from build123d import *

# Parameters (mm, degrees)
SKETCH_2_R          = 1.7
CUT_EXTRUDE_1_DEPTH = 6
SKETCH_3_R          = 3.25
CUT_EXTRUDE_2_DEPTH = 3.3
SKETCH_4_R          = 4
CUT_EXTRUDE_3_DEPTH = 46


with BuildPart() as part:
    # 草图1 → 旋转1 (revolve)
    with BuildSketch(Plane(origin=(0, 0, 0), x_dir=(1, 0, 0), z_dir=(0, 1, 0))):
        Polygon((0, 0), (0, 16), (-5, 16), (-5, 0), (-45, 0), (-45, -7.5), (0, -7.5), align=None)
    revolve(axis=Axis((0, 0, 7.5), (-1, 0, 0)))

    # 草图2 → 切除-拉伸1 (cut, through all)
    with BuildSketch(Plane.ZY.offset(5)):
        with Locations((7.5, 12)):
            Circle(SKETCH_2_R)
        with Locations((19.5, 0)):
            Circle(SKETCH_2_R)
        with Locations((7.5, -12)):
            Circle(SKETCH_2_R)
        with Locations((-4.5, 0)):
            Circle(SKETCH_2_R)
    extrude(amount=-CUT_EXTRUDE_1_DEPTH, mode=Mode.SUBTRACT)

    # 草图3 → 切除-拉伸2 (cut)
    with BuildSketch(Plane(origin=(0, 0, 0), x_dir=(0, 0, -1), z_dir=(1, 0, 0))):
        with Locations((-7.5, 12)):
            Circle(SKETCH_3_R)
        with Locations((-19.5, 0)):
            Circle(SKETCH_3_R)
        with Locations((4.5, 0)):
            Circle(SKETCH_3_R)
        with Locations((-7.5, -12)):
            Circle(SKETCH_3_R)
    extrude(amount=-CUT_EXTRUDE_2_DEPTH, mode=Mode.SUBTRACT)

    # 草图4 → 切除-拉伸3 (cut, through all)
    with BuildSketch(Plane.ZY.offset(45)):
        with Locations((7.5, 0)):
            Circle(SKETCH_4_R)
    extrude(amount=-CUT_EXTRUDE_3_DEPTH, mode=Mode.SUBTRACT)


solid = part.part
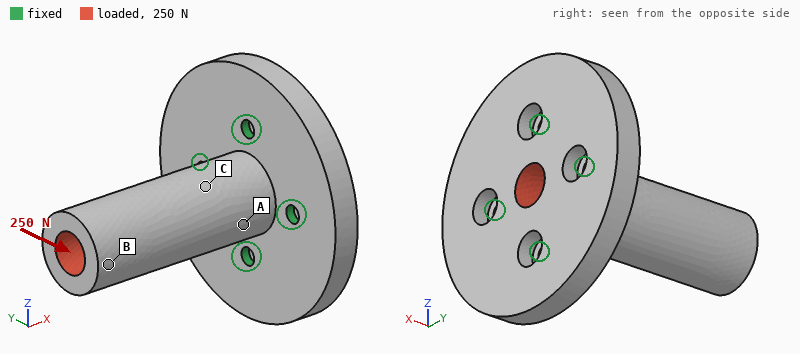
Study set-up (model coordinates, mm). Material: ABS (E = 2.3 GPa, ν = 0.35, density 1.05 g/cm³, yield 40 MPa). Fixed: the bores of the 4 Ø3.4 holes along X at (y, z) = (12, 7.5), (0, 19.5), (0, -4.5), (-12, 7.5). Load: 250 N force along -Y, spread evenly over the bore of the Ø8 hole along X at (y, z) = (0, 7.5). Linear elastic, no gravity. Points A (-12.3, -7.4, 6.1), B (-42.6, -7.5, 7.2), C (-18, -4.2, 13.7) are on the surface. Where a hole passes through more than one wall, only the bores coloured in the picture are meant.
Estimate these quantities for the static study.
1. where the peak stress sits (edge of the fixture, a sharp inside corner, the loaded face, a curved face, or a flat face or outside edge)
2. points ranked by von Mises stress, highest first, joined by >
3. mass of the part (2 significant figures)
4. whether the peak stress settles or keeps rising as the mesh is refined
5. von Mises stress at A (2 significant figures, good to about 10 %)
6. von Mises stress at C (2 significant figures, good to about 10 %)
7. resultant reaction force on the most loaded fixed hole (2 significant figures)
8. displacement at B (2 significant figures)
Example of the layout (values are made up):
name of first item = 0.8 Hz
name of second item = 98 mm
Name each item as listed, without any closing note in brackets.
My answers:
where the peak stress sits = edge of the fixture
points ranked by von Mises stress, highest first, joined by > = A > C > B
mass of the part = 14 g
whether the peak stress settles or keeps rising as the mesh is refined = keeps rising
von Mises stress at A = 9.1 MPa
von Mises stress at C = 4.6 MPa
resultant reaction force on the most loaded fixed hole = 200 N
displacement at B = 0.76 mm
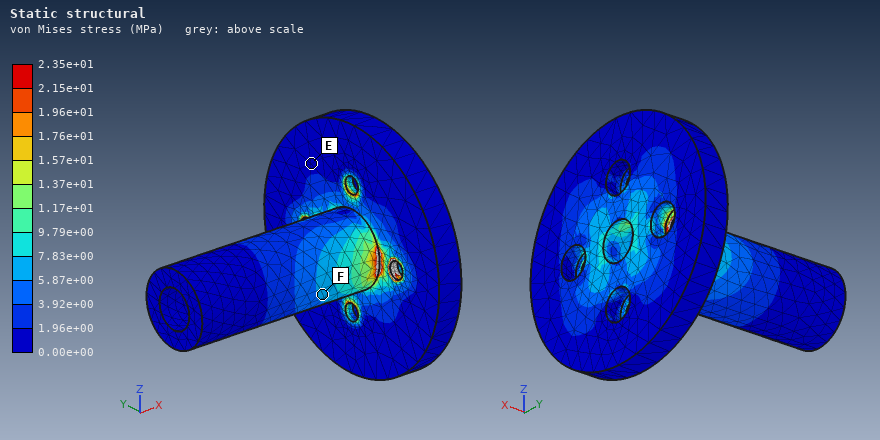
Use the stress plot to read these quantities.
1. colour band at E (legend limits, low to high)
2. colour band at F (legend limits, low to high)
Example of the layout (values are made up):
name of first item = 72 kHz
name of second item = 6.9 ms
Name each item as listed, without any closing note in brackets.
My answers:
colour band at E = 0.00e+00 to 1.96e+00 MPa
colour band at F = 5.87e+00 to 7.83e+00 MPa
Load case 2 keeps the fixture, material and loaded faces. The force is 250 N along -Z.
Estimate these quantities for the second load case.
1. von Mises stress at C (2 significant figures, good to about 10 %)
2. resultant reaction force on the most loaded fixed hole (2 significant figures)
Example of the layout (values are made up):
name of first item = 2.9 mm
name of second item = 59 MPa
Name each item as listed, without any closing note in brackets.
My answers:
von Mises stress at C = 5.7 MPa
resultant reaction force on the most loaded fixed hole = 200 N
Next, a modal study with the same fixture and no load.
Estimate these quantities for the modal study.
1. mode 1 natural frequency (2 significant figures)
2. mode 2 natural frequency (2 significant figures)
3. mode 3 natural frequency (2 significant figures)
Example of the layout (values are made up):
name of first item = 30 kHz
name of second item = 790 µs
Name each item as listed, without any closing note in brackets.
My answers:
mode 1 natural frequency = 1400 Hz
mode 2 natural frequency = 1400 Hz
mode 3 natural frequency = 3900 Hz
